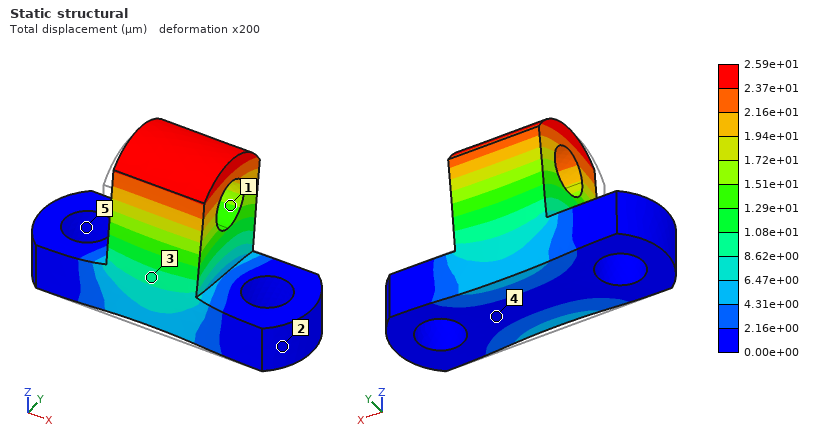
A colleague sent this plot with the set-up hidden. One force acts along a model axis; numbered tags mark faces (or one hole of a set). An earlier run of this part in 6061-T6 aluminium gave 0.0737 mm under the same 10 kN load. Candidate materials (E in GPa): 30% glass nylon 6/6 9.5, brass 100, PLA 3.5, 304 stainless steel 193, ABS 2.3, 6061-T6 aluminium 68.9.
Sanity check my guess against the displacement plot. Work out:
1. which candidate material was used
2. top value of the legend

304 stainless steel
2.59e+01 µm
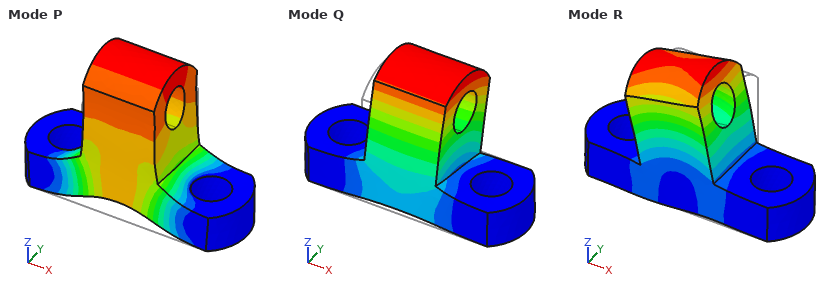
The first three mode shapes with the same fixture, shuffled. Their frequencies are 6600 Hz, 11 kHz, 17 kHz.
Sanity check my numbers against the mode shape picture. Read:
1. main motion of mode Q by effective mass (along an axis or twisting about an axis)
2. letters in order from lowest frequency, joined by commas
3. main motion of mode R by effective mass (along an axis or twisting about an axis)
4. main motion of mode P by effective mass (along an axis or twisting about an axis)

along Y
Q, R, P
along X
along Z
